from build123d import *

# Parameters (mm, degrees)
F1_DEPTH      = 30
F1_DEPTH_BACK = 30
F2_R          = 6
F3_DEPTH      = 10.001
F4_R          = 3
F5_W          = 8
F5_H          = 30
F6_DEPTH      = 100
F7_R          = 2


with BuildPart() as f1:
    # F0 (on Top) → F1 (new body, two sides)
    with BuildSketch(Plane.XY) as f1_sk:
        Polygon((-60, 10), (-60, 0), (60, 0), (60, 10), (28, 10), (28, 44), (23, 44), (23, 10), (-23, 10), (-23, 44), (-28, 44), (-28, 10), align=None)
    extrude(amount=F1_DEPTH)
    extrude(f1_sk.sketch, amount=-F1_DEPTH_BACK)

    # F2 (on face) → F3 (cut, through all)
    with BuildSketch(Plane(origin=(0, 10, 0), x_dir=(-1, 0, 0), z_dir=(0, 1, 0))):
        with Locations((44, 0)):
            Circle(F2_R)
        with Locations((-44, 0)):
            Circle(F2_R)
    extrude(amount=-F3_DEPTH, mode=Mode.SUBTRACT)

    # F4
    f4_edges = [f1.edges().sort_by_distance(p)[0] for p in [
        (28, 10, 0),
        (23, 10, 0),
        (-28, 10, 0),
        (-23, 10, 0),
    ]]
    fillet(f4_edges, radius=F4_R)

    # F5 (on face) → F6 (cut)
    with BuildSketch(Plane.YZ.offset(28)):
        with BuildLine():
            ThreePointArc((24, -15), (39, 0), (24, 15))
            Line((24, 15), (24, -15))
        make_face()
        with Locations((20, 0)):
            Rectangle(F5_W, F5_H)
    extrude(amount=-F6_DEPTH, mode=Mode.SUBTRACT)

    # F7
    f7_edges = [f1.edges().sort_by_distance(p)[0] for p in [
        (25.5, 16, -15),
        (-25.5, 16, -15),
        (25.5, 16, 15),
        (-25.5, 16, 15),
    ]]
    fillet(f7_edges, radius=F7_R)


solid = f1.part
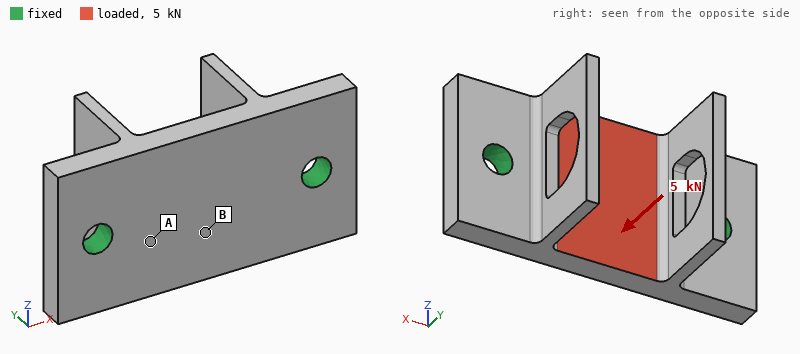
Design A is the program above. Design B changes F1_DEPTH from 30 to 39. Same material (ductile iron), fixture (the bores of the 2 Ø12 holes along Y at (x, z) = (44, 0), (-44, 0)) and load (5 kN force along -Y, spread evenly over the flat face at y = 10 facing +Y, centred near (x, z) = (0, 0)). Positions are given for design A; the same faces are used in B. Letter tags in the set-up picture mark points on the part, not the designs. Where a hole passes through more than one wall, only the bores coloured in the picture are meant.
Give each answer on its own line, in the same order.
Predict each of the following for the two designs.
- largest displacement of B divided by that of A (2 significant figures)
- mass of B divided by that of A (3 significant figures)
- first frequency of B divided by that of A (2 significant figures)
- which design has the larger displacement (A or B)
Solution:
1.1
1.16
1.0
B
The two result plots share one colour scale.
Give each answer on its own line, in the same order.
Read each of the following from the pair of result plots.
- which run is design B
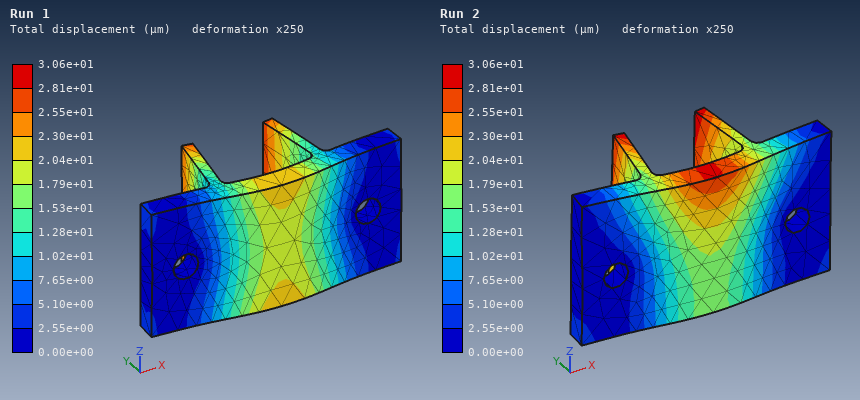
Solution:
Run 2
